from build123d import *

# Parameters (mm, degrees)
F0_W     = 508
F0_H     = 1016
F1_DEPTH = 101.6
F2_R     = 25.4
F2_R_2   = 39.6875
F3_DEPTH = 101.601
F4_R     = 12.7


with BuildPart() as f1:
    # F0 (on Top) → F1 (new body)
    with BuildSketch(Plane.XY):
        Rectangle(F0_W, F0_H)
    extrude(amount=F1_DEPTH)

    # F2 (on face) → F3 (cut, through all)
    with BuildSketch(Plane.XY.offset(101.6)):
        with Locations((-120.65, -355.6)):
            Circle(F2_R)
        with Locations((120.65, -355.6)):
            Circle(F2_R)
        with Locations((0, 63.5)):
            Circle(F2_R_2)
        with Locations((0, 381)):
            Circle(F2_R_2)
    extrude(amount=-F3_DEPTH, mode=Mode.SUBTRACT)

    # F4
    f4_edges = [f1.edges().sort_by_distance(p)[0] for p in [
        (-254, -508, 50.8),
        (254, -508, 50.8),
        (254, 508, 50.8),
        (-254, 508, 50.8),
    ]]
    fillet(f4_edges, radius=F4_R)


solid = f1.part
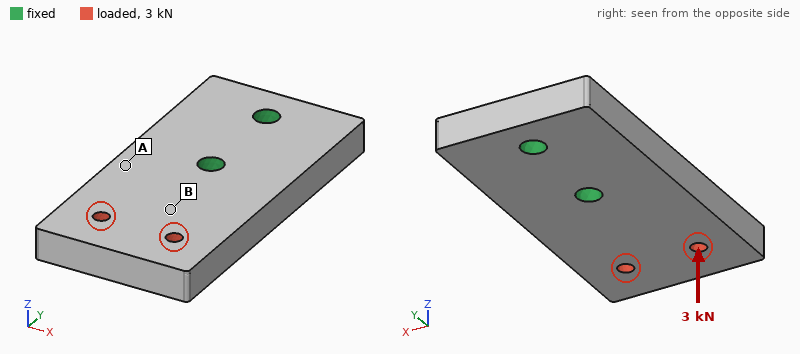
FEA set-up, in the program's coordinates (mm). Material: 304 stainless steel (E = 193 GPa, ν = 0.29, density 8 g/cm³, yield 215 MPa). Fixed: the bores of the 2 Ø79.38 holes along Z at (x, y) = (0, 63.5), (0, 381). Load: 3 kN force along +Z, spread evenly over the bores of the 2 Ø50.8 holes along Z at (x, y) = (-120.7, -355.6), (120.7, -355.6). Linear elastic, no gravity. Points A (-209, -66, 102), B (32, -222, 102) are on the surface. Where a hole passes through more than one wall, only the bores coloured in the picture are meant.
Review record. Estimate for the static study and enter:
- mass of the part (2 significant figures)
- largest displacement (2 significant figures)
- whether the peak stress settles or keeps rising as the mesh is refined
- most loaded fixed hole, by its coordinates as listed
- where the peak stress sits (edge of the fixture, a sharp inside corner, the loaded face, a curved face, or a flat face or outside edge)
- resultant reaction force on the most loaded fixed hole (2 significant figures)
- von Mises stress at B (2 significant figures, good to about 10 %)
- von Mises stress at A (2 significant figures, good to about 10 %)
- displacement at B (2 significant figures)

410 kg
15 µm
keeps rising
(0, 63.5)
edge of the fixture
4.4 kN
0.41 MPa
0.84 MPa
5.7 µm
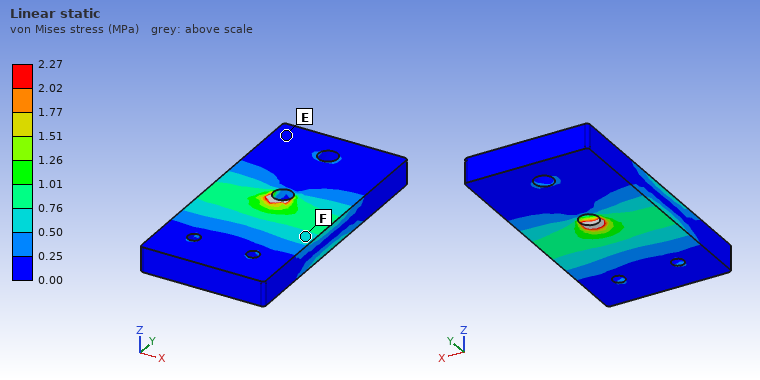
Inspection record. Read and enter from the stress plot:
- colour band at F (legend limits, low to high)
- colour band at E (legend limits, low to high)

0.50 to 0.76 MPa
0.00 to 0.25 MPa
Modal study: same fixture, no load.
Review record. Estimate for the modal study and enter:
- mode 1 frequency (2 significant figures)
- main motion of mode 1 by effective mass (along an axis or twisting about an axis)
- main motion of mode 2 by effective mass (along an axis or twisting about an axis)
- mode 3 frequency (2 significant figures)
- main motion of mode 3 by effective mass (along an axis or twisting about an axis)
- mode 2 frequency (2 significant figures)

230 Hz
along Z
twisting about Y
590 Hz
along X
480 Hz
